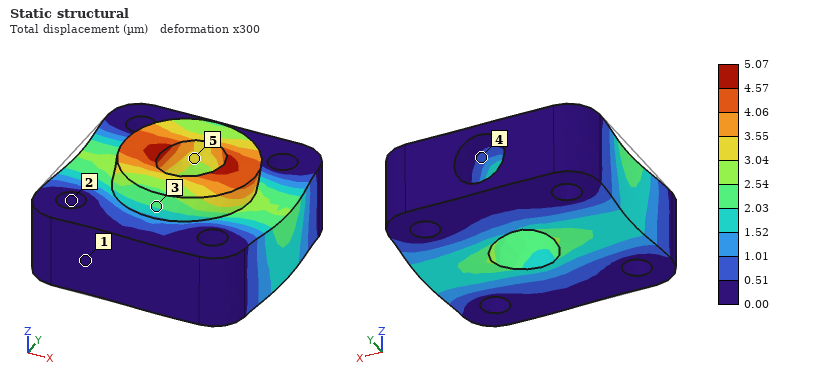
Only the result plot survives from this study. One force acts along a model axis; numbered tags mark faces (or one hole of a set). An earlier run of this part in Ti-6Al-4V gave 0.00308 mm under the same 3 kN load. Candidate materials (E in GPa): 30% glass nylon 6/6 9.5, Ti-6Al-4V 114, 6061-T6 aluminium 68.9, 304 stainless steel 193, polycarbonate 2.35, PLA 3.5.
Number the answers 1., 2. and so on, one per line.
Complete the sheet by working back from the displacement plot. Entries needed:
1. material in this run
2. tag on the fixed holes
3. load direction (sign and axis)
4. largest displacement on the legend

1. 6061-T6 aluminium
2. 2
3. +X
4. 5.07 µm
